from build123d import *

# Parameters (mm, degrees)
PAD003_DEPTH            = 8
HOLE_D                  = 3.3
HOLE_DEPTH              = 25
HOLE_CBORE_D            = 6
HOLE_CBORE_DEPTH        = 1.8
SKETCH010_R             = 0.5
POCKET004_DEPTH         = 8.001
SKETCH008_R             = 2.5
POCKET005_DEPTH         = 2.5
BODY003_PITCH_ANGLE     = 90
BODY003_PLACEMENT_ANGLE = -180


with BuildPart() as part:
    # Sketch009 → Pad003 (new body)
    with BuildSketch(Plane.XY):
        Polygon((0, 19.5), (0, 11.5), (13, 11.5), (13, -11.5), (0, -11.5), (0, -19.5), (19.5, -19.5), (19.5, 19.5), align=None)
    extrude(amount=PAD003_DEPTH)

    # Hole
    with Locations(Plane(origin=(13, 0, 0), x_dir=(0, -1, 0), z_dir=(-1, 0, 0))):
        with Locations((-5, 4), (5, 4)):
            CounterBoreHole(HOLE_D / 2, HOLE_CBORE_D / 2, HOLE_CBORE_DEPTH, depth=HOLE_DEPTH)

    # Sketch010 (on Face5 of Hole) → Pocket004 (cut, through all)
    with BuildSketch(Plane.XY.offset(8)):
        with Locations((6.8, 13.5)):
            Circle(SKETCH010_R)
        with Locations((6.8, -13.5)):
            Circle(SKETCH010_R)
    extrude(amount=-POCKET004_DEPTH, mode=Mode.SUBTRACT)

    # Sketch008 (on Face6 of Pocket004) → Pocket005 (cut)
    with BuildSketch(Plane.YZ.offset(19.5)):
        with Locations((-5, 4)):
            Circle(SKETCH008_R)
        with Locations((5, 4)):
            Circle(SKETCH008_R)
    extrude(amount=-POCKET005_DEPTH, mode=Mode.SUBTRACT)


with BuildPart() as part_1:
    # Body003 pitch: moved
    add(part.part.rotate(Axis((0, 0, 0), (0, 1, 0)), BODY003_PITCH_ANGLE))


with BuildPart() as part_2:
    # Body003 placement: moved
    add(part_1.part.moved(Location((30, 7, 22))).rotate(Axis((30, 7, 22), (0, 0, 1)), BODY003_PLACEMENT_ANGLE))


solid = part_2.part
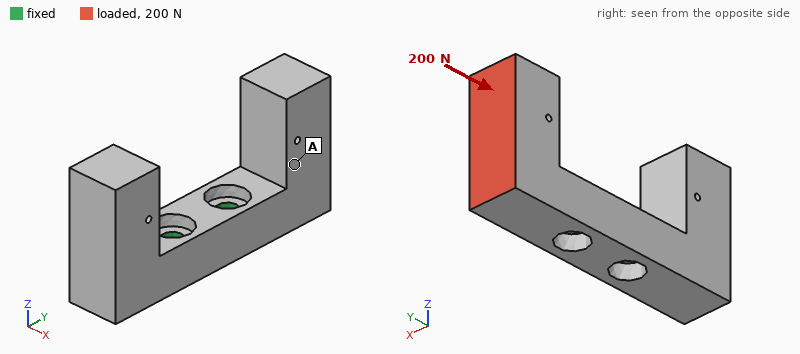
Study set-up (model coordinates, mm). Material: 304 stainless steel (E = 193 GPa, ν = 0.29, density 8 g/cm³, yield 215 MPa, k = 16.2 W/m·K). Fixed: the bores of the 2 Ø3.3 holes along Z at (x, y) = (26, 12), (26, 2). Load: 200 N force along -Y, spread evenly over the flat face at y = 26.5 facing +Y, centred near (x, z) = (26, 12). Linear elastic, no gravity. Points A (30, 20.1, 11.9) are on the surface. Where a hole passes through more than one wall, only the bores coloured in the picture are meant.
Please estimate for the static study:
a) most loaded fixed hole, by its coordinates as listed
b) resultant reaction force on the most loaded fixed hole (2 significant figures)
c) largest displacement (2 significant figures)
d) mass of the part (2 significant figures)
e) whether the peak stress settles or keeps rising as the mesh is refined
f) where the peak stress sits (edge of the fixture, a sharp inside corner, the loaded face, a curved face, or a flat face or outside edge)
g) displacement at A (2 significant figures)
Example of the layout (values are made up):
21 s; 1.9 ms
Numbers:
(26, 12); 220 N; 14 µm; 28 g; keeps rising; edge of the fixture; 5.5 µm
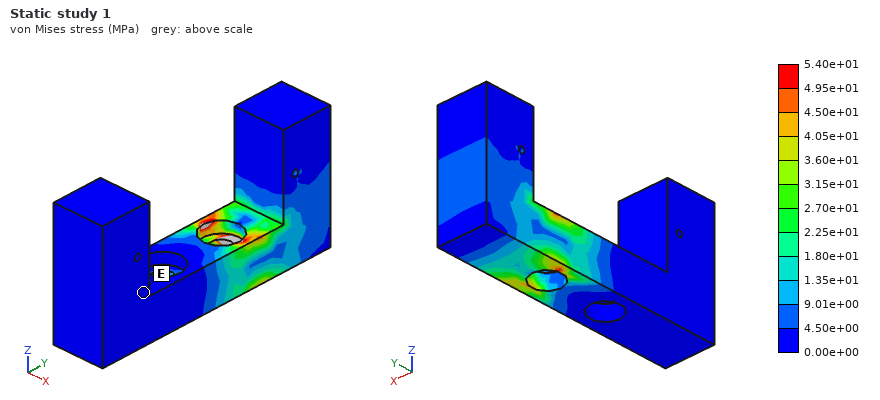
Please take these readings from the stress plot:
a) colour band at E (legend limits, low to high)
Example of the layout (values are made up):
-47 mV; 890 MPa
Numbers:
0.00e+00 to 4.50e+00 MPa
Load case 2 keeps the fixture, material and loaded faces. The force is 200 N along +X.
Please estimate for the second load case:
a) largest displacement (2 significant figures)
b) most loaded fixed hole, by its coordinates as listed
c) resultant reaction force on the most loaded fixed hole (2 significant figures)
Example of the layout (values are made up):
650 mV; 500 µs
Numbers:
19 µm; (26, 12); 360 N
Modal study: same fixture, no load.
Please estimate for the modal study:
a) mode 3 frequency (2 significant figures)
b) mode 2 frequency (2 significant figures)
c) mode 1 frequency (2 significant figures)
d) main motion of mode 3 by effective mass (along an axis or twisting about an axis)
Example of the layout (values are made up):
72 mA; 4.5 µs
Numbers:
6700 Hz; 5800 Hz; 5800 Hz; along X
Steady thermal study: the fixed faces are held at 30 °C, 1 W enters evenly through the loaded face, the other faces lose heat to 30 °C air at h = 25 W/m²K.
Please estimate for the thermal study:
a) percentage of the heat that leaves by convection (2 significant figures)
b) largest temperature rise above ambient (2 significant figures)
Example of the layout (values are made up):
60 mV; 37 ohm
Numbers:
21 %; 16 K
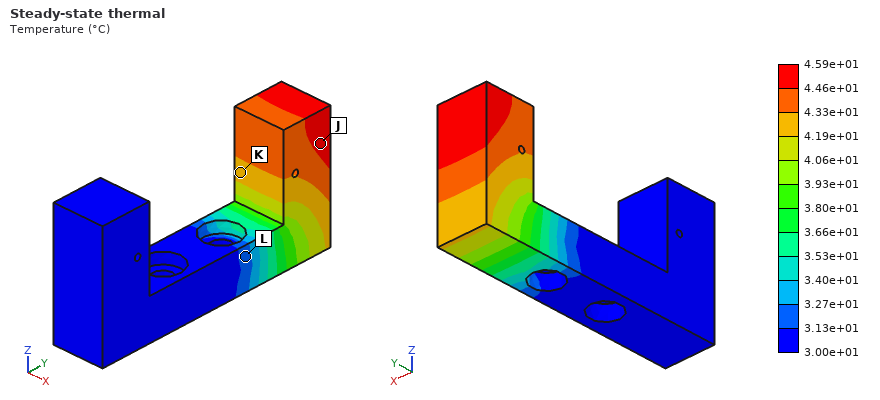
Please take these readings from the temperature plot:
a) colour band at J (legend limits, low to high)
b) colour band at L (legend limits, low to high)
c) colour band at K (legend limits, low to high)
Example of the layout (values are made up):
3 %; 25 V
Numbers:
4.46e+01 to 4.59e+01 °C; 3.13e+01 to 3.27e+01 °C; 4.19e+01 to 4.33e+01 °C
